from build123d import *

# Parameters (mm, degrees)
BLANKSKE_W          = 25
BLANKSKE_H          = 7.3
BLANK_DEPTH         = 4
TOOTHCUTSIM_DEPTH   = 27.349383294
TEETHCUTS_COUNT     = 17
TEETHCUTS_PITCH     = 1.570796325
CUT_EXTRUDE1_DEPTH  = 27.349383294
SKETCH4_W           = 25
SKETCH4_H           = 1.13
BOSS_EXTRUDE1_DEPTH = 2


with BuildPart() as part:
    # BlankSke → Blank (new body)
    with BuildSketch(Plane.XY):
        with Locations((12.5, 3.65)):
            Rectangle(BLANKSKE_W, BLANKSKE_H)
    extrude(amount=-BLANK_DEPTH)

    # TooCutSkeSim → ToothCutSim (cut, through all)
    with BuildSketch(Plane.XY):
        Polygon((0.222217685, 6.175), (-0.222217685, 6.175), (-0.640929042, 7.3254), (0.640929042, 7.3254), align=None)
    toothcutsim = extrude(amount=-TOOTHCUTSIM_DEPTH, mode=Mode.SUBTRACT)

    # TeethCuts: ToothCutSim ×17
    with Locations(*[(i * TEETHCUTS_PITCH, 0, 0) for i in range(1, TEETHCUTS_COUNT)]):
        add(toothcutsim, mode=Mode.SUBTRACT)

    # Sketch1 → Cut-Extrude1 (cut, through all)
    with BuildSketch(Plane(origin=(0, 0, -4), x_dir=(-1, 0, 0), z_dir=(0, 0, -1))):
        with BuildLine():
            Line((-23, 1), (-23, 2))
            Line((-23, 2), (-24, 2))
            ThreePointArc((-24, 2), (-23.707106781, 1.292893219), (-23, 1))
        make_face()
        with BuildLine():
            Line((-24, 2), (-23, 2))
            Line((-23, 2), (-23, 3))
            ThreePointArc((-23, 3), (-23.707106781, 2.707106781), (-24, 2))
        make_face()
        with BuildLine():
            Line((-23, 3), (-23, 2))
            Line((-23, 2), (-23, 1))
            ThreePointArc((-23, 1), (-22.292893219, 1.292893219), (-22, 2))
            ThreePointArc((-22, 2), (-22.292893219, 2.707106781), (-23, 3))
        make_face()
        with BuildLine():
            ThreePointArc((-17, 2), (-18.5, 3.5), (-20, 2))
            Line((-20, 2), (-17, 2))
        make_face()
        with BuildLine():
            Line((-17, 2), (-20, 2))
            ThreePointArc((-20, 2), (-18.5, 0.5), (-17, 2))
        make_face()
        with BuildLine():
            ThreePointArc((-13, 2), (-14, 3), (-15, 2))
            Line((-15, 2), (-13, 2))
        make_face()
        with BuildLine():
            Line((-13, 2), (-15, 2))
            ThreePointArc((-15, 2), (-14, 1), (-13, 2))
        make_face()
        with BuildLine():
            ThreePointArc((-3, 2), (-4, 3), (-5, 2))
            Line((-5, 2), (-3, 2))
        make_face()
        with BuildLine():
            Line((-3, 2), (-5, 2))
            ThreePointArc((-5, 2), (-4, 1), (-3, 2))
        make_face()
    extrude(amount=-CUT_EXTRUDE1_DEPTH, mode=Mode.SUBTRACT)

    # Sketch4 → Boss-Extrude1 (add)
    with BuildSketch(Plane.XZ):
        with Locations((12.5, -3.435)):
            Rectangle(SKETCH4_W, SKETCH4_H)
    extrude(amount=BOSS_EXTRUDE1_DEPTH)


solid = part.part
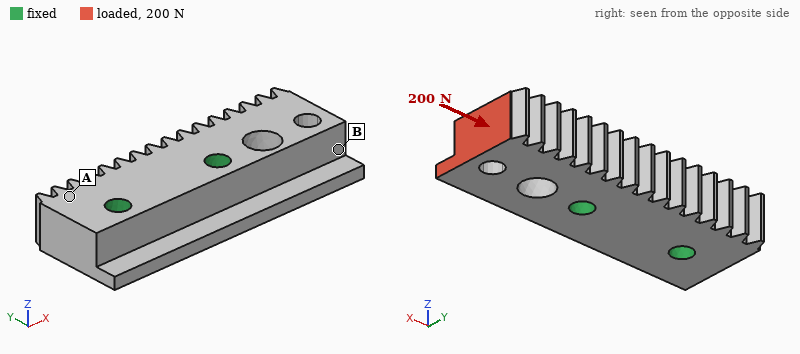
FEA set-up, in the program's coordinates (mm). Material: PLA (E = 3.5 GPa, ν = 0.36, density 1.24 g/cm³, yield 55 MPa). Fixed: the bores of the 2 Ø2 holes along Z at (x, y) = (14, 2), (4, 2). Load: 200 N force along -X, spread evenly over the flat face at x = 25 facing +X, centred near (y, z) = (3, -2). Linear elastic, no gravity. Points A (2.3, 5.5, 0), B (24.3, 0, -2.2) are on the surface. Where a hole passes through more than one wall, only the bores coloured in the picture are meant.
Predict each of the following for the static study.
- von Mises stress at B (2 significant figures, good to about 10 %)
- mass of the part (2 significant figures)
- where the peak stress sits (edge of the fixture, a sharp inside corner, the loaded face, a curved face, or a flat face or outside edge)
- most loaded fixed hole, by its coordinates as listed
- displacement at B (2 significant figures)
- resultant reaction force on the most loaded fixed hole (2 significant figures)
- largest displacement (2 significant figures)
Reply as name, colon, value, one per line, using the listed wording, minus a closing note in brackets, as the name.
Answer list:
von Mises stress at B: 7.6 MPa
mass of the part: 0.82 g
where the peak stress sits: a curved face
most loaded fixed hole, by its coordinates as listed: (14, 2)
displacement at B: 41 µm
resultant reaction force on the most loaded fixed hole: 170 N
largest displacement: 52 µm
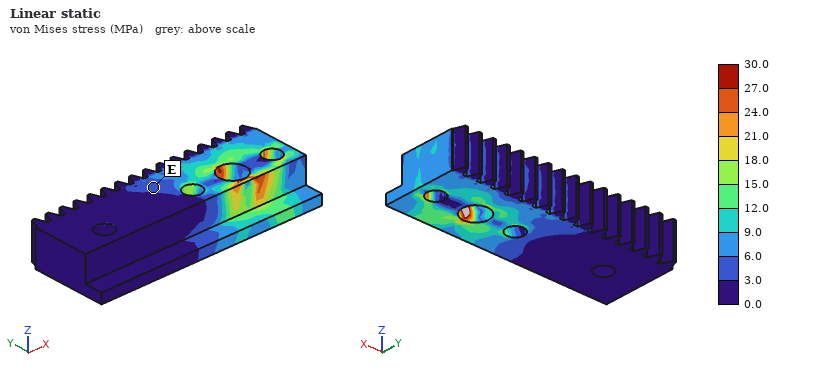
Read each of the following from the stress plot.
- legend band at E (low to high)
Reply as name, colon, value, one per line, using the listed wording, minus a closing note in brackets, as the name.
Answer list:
legend band at E: 3.0 to 6.0 MPa
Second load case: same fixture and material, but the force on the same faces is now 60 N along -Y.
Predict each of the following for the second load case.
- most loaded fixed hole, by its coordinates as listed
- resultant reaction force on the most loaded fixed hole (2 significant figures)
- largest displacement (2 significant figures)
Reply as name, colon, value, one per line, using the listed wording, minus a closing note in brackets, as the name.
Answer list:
most loaded fixed hole, by its coordinates as listed: (14, 2)
resultant reaction force on the most loaded fixed hole: 100 N
largest displacement: 0.18 mm
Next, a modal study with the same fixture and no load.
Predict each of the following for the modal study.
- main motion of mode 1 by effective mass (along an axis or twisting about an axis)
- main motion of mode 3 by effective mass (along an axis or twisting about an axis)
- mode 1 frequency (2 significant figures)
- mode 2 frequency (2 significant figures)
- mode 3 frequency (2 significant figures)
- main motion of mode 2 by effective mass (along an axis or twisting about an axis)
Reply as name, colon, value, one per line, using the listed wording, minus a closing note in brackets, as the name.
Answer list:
main motion of mode 1 by effective mass: along Z
main motion of mode 3 by effective mass: twisting about X
mode 1 frequency: 7100 Hz
mode 2 frequency: 9300 Hz
mode 3 frequency: 14 kHz
main motion of mode 2 by effective mass: along Y
